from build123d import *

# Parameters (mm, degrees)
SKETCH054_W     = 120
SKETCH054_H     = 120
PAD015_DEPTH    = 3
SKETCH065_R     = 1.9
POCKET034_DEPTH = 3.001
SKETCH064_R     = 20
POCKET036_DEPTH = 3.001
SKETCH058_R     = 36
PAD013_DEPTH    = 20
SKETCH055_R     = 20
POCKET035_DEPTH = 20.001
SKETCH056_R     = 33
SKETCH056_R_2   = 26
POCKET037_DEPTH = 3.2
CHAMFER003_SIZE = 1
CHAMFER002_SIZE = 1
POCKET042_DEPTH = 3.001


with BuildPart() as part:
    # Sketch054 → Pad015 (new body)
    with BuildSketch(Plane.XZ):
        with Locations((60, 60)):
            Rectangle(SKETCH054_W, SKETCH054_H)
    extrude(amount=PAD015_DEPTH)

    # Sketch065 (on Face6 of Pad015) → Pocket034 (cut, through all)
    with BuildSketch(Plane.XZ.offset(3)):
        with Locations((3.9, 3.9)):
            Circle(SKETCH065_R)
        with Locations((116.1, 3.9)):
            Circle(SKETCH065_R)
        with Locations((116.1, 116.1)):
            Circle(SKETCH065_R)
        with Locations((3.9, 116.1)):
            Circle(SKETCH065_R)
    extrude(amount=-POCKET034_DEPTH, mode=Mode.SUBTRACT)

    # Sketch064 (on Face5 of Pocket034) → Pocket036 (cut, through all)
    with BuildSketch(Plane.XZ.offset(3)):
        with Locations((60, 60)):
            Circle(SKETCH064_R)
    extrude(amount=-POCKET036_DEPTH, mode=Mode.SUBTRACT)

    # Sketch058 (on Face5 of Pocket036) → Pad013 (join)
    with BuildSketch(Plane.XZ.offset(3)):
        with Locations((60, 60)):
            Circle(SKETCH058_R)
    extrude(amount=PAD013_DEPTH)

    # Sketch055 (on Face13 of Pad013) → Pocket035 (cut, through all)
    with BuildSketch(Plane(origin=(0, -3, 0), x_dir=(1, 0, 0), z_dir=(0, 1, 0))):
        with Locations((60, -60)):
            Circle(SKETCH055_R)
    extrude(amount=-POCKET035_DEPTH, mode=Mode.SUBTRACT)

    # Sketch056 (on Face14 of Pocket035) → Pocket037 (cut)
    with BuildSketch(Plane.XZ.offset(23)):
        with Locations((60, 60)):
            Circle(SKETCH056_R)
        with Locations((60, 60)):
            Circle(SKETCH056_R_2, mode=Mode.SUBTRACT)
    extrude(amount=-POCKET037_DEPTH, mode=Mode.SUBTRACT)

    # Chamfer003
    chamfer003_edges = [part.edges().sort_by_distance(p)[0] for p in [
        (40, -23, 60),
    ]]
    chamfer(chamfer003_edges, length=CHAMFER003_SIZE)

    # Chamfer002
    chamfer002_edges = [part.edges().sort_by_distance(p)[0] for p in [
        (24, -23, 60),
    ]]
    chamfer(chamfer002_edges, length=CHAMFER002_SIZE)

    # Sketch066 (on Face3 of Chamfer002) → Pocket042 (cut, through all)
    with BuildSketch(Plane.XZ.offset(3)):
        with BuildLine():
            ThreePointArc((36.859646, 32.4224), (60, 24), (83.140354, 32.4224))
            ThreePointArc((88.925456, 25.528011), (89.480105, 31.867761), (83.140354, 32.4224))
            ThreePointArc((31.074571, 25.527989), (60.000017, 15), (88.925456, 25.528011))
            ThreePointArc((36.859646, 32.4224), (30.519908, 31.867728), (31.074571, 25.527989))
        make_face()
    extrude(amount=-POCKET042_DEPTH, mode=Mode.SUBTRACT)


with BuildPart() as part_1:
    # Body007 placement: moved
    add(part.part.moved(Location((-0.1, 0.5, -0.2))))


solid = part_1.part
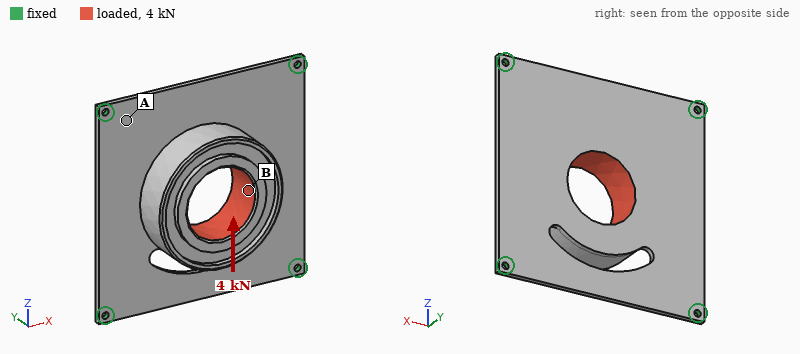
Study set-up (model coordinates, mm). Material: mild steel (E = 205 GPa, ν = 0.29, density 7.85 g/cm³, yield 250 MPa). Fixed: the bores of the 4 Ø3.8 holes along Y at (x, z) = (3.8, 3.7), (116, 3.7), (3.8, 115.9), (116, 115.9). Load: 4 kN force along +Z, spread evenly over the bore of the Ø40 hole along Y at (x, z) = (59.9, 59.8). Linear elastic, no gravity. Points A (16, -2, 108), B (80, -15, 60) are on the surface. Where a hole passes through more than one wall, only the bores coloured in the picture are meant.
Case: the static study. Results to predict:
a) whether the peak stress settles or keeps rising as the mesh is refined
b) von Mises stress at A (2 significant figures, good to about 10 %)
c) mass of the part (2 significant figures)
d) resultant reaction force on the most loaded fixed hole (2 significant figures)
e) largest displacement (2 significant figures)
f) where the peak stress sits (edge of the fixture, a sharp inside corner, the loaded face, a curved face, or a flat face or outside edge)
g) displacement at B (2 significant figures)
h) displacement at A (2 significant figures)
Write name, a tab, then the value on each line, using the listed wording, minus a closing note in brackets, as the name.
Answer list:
whether the peak stress settles or keeps rising as the mesh is refined	keeps rising
von Mises stress at A	37 MPa
mass of the part	700 g
resultant reaction force on the most loaded fixed hole	1.2 kN
largest displacement	0.16 mm
where the peak stress sits	edge of the fixture
displacement at B	0.058 mm
displacement at A	0.024 mm
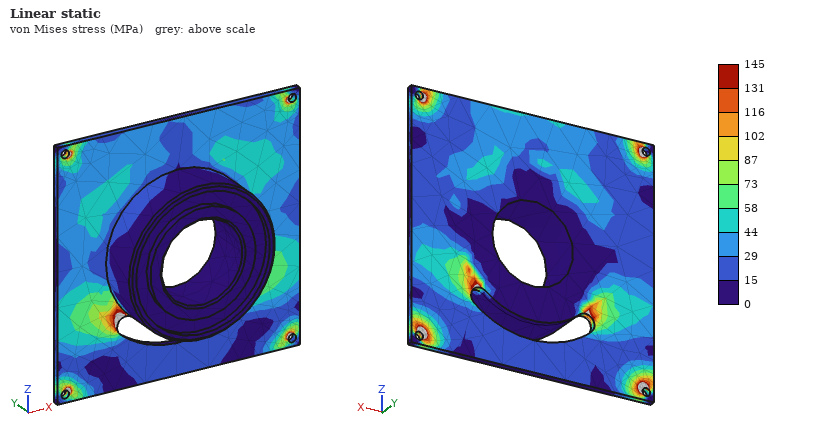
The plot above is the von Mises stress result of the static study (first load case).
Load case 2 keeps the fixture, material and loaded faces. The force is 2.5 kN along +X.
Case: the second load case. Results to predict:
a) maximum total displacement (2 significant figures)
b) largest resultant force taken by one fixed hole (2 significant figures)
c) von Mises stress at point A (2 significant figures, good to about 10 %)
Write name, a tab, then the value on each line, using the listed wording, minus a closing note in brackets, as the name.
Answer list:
maximum total displacement	73 µm
largest resultant force taken by one fixed hole	990 N
von Mises stress at point A	26 MPa
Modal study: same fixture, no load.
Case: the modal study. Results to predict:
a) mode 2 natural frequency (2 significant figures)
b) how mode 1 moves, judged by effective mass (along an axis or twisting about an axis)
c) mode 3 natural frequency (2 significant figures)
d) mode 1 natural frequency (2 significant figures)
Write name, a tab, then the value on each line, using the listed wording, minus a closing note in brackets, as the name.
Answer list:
mode 2 natural frequency	990 Hz
how mode 1 moves, judged by effective mass	along Y
mode 3 natural frequency	1000 Hz
mode 1 natural frequency	530 Hz
